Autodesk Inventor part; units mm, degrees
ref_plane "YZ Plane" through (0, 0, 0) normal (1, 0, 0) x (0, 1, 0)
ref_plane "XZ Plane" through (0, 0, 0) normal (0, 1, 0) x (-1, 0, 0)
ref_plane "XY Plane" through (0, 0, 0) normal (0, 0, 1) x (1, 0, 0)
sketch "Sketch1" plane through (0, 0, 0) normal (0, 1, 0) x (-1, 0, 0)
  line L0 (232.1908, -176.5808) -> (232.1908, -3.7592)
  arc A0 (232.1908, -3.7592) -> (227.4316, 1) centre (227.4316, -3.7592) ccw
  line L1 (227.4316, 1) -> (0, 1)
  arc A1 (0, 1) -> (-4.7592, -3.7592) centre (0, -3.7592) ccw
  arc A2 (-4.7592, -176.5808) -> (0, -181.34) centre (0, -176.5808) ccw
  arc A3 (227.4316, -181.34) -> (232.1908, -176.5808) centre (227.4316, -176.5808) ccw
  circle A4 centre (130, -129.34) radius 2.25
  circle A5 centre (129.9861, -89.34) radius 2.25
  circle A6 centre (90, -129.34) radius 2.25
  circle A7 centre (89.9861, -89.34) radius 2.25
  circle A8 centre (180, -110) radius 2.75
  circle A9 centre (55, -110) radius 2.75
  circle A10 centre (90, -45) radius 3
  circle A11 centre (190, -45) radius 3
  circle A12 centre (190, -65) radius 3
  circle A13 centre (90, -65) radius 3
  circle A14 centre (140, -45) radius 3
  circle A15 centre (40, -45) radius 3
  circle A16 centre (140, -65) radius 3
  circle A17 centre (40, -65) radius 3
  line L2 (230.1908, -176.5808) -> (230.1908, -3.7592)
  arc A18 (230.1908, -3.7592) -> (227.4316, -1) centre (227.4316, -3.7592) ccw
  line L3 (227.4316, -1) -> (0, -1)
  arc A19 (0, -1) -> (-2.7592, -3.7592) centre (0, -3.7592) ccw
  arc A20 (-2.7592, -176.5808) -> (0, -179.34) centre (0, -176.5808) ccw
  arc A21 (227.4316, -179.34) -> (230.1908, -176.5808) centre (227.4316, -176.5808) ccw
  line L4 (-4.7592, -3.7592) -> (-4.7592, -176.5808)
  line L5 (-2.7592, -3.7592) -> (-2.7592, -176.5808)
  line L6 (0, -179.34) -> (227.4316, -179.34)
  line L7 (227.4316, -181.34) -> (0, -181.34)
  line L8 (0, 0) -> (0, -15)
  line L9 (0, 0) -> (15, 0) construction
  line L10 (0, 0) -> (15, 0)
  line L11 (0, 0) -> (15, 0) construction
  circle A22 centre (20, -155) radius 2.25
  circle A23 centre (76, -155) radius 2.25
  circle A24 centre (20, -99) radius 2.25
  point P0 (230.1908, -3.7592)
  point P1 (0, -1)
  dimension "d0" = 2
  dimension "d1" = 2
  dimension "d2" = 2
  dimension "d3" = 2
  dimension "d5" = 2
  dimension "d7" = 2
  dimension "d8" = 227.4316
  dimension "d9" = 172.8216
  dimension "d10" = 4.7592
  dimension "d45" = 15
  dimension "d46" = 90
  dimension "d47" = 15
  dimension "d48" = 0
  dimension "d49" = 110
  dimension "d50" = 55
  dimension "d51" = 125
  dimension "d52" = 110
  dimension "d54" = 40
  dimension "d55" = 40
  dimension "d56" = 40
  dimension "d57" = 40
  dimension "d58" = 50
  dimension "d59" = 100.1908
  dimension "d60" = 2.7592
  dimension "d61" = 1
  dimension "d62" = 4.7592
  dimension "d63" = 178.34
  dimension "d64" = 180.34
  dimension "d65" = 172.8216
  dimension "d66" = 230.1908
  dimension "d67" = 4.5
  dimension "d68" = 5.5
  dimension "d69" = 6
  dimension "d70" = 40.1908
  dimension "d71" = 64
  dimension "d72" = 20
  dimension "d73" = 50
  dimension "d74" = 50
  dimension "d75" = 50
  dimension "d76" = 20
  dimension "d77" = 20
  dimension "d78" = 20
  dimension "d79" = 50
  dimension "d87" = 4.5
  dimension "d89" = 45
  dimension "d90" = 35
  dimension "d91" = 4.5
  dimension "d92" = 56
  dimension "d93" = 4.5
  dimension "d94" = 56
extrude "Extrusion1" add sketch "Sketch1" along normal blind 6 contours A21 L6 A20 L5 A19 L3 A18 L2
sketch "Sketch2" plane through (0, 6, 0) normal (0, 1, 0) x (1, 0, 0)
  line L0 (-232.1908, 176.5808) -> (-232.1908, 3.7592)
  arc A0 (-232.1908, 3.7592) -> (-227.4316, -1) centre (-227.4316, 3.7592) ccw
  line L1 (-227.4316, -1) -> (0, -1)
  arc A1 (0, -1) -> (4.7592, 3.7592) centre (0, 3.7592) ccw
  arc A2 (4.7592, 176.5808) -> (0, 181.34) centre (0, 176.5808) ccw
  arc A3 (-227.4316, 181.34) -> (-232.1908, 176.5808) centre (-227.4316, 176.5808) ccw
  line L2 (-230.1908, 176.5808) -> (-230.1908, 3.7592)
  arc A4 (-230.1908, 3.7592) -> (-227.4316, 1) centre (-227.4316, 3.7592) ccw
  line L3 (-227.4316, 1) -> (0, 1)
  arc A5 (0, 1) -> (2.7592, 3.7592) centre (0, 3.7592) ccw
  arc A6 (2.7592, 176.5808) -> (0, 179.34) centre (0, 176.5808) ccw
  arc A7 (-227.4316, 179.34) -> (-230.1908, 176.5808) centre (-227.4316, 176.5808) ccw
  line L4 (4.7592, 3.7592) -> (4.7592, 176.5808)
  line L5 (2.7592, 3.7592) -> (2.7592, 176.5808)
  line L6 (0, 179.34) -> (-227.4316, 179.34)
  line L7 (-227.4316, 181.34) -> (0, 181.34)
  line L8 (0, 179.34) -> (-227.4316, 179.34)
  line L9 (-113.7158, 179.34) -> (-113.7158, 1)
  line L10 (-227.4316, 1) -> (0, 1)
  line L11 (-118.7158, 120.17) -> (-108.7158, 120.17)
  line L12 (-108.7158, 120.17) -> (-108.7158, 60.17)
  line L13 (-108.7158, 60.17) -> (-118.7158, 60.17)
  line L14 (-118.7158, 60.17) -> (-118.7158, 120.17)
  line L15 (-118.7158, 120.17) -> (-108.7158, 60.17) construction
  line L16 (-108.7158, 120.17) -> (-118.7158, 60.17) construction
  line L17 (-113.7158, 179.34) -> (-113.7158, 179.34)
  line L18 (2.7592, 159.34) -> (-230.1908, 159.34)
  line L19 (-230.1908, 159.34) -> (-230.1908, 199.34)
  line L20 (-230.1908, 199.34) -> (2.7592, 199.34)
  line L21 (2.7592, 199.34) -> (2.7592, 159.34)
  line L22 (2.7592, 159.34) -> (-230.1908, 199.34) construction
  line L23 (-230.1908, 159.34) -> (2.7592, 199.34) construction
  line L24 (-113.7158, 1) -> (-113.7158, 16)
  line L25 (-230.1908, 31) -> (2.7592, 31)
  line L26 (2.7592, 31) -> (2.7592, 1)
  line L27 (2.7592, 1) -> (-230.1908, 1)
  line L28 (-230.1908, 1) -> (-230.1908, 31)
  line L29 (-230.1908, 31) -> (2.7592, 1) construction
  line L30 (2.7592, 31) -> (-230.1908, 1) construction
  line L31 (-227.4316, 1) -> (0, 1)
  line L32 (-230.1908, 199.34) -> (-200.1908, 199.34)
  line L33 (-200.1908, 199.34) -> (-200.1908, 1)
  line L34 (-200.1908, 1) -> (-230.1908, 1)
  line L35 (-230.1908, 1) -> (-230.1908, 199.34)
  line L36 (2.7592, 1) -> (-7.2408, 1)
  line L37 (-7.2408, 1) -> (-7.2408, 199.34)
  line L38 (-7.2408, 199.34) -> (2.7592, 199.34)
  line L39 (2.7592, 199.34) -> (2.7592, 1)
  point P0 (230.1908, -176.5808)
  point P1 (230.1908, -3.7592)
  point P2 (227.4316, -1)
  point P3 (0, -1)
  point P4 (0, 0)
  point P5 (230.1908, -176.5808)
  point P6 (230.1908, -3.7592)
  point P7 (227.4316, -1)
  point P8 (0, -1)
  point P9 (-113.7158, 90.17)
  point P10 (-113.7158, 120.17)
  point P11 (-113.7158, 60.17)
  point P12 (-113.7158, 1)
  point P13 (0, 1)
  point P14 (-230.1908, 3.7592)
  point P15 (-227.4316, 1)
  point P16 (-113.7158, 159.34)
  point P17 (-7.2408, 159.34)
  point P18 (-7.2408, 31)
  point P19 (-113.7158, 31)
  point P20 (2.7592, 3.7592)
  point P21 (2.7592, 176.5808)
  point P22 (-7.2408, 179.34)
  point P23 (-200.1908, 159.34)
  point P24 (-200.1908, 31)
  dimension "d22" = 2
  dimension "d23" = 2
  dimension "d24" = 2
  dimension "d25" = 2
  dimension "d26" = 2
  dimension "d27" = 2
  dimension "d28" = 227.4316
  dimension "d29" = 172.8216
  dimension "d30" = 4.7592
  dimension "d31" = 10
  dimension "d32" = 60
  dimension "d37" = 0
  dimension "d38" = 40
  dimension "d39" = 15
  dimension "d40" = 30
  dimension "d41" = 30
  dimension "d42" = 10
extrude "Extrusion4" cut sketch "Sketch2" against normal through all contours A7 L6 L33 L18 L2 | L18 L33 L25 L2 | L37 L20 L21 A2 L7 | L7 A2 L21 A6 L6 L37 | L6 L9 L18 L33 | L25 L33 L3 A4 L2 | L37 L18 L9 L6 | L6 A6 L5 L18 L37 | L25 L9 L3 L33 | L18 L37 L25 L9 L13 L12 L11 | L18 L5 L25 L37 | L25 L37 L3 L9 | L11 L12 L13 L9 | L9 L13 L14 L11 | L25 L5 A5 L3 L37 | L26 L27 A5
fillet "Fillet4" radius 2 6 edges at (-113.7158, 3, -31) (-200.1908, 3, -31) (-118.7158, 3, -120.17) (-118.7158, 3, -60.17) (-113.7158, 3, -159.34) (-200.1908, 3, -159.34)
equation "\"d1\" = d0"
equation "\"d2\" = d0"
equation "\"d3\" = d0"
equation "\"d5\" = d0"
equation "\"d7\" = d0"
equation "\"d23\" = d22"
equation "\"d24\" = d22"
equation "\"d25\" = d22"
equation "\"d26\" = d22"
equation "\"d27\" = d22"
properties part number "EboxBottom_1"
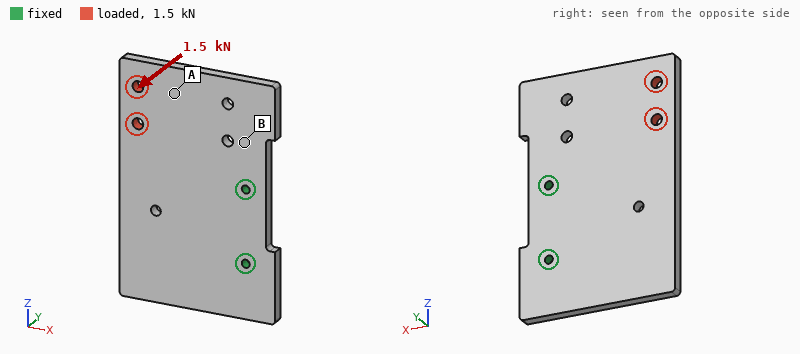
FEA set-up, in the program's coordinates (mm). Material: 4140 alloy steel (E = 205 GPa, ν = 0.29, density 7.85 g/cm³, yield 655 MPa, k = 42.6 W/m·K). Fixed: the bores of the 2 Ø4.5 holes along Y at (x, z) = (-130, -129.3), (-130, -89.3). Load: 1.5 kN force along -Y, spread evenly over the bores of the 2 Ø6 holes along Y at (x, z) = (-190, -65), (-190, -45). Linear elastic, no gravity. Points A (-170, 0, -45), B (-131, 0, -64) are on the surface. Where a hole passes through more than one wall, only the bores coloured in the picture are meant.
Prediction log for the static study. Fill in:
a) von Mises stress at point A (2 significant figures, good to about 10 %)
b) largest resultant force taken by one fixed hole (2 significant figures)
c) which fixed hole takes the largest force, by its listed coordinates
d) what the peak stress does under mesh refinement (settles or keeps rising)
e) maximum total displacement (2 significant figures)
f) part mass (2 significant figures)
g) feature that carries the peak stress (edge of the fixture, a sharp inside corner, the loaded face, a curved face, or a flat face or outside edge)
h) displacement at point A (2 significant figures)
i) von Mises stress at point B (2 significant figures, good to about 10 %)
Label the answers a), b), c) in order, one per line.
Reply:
a) 49 MPa
b) 2.2 kN
c) (-130, -89.3)
d) keeps rising
e) 0.99 mm
f) 500 g
g) edge of the fixture
h) 0.54 mm
i) 130 MPa
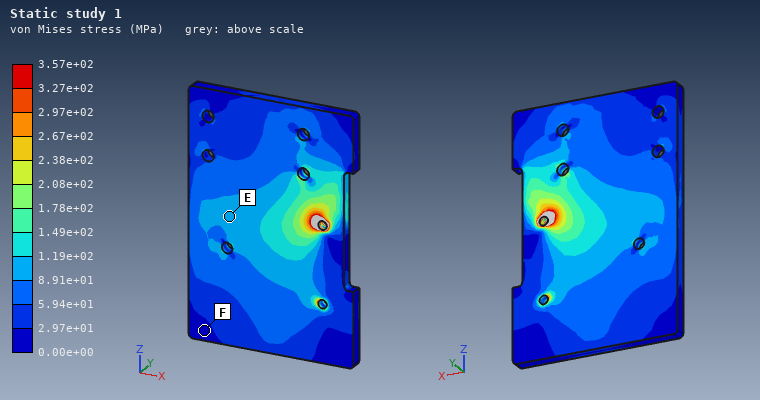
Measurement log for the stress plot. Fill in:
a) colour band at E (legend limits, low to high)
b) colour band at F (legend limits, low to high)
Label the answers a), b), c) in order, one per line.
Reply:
a) 8.91e+01 to 1.19e+02 MPa
b) 0.00e+00 to 2.97e+01 MPa
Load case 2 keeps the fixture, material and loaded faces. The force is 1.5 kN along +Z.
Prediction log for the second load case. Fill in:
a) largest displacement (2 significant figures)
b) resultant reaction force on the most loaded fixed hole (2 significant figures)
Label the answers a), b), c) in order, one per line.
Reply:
a) 16 µm
b) 2.3 kN
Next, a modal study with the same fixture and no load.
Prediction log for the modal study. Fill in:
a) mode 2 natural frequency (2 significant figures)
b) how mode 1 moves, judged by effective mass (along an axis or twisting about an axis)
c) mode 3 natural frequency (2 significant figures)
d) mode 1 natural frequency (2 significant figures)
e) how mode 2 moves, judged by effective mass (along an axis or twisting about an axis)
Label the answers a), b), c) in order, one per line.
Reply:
a) 1100 Hz
b) along Y
c) 1800 Hz
d) 740 Hz
e) twisting about X
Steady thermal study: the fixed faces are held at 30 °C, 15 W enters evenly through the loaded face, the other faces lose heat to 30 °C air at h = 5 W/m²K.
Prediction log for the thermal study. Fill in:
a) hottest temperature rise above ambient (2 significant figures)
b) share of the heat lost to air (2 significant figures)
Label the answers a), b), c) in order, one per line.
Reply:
a) 67 K
b) 18 %
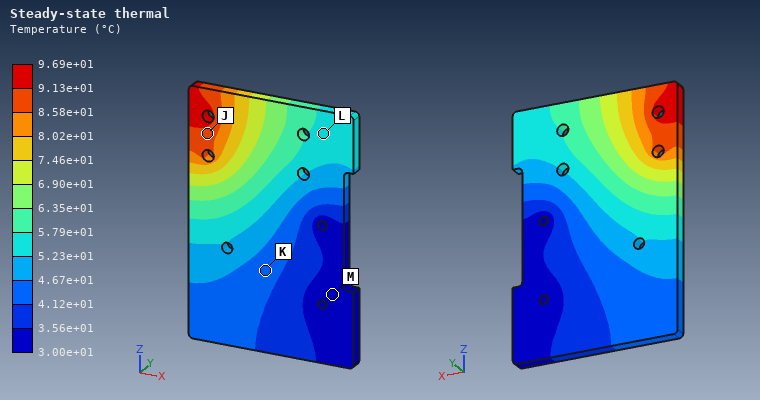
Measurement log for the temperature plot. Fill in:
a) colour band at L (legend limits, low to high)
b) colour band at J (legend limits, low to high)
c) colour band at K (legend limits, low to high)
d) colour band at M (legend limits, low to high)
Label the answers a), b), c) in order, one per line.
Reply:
a) 5.23e+01 to 5.79e+01 °C
b) 8.58e+01 to 9.13e+01 °C
c) 4.12e+01 to 4.67e+01 °C
d) 3.00e+01 to 3.56e+01 °C
